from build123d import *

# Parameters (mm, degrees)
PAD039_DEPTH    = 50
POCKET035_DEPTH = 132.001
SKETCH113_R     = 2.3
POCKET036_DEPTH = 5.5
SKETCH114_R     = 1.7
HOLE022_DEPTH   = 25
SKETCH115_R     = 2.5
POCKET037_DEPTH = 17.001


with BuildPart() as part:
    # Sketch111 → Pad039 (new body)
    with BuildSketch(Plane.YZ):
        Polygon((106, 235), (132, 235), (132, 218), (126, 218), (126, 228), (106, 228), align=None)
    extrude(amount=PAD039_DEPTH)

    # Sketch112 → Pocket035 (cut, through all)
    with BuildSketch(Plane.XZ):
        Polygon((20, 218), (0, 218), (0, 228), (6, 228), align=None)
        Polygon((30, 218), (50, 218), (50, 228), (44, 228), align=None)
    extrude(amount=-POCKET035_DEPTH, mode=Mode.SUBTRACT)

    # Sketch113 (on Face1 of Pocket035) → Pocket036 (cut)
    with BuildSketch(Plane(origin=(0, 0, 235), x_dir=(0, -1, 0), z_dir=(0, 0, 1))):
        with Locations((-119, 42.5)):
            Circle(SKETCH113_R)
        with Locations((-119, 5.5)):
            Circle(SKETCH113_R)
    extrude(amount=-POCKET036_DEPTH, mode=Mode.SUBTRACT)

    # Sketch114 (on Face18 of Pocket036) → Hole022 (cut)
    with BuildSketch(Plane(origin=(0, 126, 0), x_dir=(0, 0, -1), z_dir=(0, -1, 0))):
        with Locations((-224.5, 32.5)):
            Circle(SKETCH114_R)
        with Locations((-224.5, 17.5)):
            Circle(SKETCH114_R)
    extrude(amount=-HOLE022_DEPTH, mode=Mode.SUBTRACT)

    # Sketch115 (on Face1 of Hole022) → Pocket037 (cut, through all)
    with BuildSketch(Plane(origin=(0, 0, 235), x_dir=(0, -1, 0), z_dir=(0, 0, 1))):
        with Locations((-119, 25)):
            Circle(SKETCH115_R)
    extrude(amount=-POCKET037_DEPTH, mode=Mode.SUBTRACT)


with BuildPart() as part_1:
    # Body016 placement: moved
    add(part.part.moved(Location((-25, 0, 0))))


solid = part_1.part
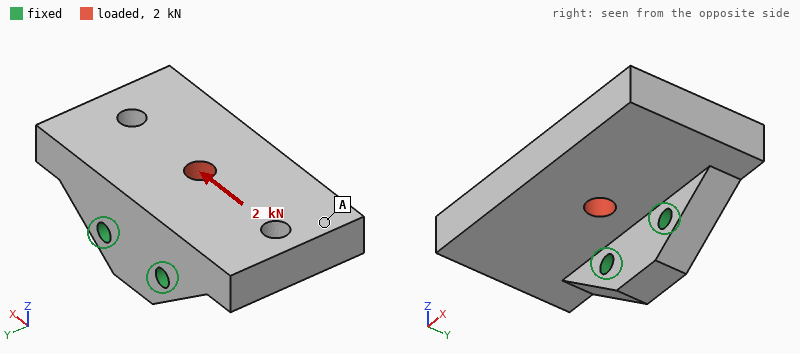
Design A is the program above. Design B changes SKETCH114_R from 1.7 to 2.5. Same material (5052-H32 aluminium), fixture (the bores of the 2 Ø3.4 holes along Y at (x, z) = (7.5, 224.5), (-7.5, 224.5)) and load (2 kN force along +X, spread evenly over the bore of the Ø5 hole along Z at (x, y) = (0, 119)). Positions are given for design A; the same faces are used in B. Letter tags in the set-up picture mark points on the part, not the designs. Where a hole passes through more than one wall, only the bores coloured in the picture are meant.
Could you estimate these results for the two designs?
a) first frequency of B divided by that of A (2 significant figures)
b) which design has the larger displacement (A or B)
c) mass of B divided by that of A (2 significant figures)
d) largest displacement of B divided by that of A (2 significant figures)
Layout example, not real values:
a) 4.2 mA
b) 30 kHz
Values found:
a) 1.1
b) A
c) 0.99
d) 0.78
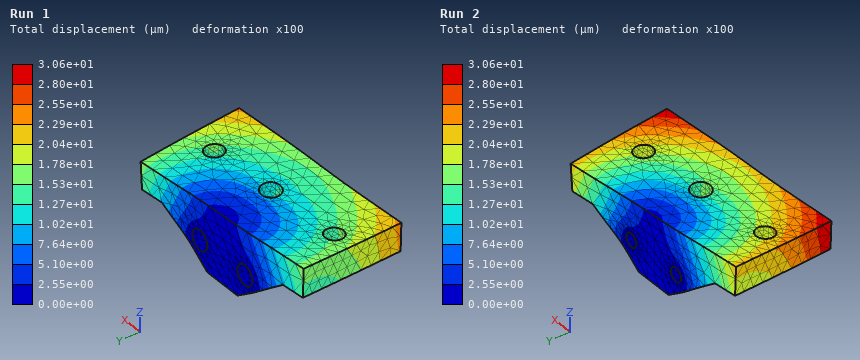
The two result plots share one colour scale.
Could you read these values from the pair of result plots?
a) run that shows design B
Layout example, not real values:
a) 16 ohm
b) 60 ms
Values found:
a) Run 1
